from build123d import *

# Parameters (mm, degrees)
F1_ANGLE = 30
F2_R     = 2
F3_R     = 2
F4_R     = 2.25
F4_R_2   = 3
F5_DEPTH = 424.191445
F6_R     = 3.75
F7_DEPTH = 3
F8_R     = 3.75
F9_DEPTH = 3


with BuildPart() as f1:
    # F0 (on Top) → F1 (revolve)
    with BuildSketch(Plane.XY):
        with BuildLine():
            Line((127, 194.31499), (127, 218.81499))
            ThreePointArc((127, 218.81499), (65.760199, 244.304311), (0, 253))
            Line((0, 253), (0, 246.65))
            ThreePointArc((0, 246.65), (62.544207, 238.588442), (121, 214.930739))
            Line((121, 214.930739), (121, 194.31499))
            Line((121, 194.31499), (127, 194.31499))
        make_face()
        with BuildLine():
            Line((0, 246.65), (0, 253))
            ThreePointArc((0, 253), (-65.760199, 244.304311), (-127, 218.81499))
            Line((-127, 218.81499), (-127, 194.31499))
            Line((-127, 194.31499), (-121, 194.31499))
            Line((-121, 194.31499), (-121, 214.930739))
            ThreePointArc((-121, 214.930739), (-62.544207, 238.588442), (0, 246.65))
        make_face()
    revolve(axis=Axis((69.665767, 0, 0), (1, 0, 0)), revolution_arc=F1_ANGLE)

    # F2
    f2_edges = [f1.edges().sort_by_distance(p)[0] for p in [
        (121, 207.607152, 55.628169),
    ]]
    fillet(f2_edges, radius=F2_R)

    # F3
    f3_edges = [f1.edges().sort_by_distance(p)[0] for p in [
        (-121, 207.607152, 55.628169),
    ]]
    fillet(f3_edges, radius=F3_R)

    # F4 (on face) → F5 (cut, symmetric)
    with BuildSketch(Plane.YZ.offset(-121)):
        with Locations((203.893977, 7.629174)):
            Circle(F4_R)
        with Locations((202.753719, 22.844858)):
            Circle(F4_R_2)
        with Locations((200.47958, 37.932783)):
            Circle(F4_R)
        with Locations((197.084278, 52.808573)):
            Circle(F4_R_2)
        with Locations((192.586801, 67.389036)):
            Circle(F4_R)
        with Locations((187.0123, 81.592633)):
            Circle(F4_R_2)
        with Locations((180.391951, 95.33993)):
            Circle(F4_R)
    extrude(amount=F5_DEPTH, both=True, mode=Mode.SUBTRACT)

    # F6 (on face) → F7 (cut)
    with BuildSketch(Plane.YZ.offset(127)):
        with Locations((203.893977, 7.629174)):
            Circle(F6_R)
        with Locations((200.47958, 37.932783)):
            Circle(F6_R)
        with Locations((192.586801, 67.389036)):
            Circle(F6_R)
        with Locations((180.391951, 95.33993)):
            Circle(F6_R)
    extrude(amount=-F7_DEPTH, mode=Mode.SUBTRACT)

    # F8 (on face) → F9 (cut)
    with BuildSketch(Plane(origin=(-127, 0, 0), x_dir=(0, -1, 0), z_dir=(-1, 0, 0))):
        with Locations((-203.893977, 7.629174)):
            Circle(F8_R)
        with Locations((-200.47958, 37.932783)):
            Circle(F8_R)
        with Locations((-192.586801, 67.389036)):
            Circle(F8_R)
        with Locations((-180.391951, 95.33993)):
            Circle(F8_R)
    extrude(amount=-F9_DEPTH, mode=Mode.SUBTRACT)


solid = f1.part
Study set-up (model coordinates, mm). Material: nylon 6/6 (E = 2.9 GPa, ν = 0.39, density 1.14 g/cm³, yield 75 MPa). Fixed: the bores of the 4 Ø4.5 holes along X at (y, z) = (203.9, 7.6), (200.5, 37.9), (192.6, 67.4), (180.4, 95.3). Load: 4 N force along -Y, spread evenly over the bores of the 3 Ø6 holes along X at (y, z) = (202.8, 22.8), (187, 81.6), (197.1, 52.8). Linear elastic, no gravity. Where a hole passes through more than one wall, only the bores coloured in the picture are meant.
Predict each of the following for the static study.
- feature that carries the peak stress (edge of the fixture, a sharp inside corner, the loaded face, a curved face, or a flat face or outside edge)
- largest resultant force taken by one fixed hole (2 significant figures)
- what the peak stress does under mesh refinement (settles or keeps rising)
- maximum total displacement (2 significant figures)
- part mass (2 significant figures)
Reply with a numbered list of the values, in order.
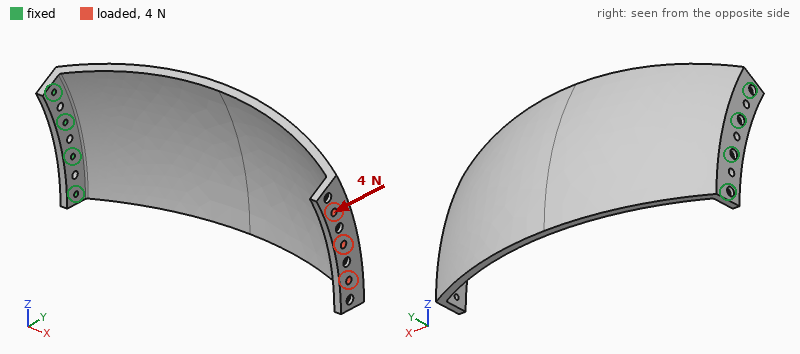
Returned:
1. edge of the fixture
2. 21 N
3. keeps rising
4. 3.1 mm
5. 270 g
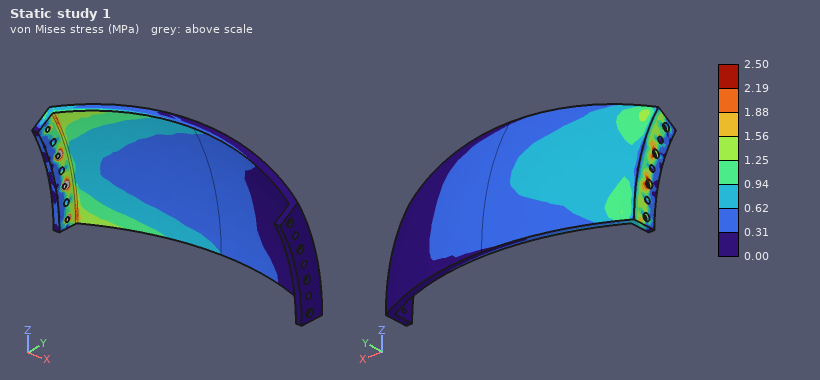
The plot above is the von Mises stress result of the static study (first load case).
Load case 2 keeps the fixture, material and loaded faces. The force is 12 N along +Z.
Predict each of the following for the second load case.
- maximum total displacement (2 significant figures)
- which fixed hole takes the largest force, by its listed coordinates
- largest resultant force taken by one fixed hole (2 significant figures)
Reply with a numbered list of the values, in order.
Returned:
1. 3.5 mm
2. (203.9, 7.6)
3. 38 N
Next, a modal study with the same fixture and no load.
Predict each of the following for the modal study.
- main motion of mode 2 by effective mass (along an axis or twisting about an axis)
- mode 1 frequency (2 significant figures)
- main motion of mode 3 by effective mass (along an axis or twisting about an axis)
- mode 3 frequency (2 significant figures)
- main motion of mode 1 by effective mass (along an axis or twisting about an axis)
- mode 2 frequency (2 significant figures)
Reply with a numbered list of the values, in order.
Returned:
1. along Z
2. 21 Hz
3. along X
4. 110 Hz
5. along Y
6. 54 Hz
